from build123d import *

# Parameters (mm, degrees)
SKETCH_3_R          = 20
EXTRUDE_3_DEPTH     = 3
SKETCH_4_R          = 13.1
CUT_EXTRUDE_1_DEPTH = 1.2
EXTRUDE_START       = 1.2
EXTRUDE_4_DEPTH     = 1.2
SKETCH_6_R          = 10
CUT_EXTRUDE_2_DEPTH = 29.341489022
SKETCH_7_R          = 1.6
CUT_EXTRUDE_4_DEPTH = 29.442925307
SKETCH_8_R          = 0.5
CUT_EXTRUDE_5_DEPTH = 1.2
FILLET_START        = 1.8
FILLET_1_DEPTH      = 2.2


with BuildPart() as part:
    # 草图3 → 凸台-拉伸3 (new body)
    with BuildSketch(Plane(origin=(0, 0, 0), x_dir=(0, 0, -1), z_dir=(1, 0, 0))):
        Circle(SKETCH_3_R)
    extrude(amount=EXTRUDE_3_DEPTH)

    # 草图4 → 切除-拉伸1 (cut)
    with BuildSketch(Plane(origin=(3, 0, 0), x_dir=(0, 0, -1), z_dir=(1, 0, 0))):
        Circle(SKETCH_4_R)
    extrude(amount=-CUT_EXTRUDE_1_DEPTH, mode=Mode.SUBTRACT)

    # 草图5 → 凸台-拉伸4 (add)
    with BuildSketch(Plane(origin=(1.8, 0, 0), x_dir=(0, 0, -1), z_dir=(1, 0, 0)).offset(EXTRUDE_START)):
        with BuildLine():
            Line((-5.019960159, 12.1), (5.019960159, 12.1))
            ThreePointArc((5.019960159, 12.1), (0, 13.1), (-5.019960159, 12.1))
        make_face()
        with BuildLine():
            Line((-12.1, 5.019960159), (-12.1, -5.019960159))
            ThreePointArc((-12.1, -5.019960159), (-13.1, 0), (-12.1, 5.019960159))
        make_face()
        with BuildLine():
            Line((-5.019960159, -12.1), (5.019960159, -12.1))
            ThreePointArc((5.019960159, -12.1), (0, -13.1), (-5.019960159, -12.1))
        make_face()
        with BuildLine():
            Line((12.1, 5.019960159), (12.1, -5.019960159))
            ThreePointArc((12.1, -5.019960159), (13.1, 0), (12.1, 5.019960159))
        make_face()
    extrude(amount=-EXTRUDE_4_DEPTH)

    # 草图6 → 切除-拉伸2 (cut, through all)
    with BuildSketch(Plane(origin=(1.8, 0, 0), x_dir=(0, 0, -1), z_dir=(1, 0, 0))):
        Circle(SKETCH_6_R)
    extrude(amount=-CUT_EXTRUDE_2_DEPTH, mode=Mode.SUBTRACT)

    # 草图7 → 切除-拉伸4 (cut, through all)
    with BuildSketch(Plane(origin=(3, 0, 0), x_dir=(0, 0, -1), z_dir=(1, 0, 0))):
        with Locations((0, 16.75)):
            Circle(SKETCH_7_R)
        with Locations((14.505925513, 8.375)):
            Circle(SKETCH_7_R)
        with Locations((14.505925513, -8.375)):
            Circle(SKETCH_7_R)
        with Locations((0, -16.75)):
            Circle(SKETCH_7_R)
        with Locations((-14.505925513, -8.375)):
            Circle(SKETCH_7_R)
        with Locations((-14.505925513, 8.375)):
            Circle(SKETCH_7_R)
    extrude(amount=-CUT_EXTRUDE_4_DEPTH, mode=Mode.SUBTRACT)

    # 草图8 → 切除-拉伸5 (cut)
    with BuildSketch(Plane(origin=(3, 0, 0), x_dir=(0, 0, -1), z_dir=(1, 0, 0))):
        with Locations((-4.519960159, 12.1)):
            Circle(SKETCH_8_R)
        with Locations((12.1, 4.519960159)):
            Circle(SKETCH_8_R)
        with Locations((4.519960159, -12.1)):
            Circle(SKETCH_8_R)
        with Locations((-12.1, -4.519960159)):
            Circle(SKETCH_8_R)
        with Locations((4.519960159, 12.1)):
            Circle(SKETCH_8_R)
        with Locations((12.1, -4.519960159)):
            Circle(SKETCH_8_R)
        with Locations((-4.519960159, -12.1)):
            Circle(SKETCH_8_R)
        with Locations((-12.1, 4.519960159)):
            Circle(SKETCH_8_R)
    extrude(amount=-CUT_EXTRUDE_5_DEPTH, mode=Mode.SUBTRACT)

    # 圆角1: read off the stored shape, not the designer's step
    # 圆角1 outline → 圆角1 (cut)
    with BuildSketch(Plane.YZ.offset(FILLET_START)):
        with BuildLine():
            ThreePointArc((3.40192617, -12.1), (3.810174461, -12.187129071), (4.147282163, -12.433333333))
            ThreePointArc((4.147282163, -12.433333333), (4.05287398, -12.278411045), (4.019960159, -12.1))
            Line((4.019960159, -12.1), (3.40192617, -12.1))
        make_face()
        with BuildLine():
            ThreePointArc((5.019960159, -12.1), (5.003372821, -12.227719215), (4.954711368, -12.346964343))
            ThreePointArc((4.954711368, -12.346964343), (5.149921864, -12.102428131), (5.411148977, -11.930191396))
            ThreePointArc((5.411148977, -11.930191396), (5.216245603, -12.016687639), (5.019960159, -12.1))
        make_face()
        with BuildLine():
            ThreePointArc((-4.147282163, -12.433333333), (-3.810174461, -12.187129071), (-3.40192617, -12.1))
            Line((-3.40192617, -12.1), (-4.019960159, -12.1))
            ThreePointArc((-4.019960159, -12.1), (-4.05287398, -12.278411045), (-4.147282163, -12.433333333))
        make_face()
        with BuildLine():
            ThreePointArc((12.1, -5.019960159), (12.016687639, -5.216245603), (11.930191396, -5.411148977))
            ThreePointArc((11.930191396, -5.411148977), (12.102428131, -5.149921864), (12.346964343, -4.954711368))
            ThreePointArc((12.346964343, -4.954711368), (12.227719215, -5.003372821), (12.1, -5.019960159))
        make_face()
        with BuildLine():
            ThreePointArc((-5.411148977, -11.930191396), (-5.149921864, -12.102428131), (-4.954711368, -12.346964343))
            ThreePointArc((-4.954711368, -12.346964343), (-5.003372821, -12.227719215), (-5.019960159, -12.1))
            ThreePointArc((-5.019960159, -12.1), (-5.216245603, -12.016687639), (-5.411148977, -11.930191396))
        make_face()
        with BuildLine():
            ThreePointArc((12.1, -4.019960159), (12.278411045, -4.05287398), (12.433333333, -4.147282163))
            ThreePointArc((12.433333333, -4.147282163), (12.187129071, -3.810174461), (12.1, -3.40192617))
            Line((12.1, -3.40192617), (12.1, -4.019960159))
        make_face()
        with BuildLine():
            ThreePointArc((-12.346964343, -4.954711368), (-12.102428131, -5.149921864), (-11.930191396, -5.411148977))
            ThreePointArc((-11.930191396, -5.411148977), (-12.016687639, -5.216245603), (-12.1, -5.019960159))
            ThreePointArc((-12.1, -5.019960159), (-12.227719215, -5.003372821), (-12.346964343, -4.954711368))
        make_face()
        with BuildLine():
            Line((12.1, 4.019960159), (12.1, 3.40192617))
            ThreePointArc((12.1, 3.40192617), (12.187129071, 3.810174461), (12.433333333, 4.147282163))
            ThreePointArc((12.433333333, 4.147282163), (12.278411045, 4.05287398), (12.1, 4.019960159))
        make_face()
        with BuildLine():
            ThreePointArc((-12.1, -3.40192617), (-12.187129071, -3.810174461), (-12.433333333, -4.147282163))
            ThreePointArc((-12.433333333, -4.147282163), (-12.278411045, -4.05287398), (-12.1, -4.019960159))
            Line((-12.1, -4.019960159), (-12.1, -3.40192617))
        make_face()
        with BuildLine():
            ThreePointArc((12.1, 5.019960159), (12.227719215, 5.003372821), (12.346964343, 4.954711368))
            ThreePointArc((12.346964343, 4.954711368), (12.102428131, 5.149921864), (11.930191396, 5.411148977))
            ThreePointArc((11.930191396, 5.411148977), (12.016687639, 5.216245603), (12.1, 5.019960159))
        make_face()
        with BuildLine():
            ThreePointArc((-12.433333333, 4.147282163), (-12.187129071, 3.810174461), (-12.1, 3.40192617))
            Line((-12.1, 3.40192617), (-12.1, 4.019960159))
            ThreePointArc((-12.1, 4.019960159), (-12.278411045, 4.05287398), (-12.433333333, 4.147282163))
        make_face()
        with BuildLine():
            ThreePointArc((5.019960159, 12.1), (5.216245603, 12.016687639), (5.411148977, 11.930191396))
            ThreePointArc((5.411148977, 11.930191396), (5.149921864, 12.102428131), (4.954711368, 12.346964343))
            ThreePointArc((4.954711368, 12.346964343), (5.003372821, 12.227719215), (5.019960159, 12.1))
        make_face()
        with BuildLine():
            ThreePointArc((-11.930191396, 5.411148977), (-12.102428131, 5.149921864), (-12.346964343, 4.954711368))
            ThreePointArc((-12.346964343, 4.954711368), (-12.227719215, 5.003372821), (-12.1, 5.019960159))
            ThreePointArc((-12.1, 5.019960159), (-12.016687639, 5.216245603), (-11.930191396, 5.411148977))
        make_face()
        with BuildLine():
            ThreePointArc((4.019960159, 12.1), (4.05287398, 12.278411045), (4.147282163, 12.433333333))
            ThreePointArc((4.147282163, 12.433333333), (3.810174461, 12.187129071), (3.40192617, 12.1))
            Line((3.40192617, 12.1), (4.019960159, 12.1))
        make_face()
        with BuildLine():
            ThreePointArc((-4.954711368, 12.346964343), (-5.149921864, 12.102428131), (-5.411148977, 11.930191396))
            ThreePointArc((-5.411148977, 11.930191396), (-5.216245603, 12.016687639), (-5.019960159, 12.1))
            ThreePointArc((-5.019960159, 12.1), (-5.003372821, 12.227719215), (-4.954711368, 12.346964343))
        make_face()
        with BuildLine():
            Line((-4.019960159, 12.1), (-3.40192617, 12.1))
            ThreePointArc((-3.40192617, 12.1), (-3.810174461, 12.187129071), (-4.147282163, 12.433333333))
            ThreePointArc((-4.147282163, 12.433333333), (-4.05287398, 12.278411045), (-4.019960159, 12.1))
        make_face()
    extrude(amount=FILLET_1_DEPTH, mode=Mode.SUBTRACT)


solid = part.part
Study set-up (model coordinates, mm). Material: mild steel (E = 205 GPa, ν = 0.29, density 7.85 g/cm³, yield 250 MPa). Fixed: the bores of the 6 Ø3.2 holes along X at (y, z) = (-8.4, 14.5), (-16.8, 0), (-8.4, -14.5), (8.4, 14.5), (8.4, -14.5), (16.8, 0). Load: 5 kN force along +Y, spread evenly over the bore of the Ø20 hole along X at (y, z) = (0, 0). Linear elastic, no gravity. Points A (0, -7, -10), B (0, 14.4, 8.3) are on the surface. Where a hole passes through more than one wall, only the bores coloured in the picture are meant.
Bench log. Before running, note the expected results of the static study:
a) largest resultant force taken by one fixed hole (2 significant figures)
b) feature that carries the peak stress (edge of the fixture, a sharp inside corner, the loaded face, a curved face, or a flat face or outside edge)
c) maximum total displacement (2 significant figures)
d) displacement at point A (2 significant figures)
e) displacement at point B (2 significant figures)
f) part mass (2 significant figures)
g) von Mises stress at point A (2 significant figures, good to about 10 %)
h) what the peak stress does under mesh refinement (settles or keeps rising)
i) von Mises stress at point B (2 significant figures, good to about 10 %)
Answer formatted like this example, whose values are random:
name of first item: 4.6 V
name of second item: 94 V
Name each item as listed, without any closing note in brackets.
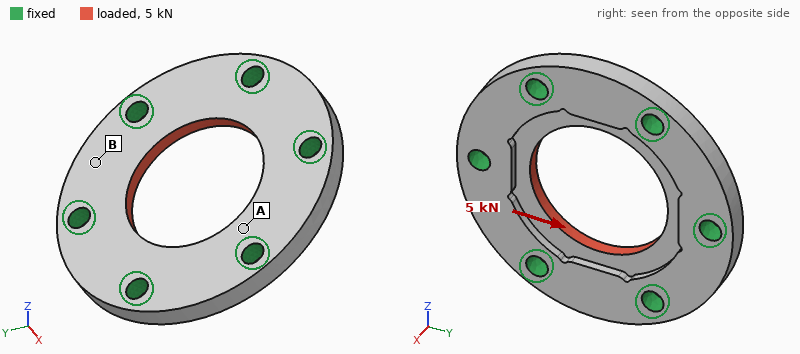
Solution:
largest resultant force taken by one fixed hole: 1.1 kN
feature that carries the peak stress: edge of the fixture
maximum total displacement: 2.9 µm
displacement at point A: 1.4 µm
displacement at point B: 1.5 µm
part mass: 19 g
von Mises stress at point A: 36 MPa
what the peak stress does under mesh refinement: keeps rising
von Mises stress at point B: 16 MPa
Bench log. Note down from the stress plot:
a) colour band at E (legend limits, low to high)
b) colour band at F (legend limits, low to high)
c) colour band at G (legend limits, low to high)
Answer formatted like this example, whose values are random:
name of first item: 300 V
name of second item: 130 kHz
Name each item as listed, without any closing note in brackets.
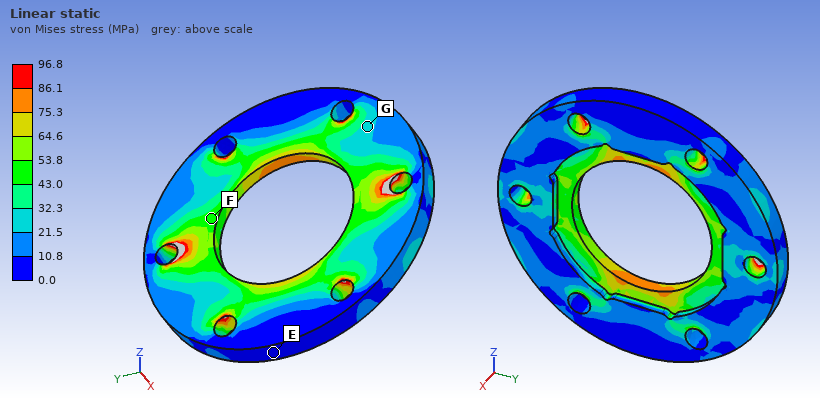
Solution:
colour band at E: 0.0 to 10.8 MPa
colour band at F: 43.0 to 53.8 MPa
colour band at G: 21.5 to 32.3 MPa
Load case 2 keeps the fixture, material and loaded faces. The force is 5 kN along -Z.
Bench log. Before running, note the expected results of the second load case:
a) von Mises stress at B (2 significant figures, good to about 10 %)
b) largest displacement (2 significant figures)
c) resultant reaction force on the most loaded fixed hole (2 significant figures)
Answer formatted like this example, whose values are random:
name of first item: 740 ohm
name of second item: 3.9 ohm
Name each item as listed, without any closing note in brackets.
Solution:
von Mises stress at B: 9.1 MPa
largest displacement: 3.2 µm
resultant reaction force on the most loaded fixed hole: 960 N
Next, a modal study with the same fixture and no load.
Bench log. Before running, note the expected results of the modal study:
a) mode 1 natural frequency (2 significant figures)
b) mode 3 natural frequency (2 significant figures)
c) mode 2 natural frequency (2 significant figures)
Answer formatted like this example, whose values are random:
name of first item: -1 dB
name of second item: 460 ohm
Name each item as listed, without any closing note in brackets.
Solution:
mode 1 natural frequency: 49 kHz
mode 3 natural frequency: 50 kHz
mode 2 natural frequency: 50 kHz
